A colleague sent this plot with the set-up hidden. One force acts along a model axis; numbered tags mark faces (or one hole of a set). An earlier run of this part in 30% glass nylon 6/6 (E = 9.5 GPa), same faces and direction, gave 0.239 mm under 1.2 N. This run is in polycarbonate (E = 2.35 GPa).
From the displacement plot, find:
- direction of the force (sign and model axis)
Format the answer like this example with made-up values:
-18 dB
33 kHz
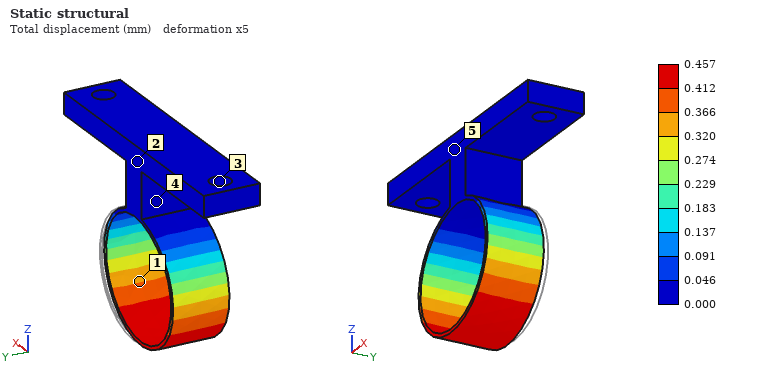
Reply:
-X
